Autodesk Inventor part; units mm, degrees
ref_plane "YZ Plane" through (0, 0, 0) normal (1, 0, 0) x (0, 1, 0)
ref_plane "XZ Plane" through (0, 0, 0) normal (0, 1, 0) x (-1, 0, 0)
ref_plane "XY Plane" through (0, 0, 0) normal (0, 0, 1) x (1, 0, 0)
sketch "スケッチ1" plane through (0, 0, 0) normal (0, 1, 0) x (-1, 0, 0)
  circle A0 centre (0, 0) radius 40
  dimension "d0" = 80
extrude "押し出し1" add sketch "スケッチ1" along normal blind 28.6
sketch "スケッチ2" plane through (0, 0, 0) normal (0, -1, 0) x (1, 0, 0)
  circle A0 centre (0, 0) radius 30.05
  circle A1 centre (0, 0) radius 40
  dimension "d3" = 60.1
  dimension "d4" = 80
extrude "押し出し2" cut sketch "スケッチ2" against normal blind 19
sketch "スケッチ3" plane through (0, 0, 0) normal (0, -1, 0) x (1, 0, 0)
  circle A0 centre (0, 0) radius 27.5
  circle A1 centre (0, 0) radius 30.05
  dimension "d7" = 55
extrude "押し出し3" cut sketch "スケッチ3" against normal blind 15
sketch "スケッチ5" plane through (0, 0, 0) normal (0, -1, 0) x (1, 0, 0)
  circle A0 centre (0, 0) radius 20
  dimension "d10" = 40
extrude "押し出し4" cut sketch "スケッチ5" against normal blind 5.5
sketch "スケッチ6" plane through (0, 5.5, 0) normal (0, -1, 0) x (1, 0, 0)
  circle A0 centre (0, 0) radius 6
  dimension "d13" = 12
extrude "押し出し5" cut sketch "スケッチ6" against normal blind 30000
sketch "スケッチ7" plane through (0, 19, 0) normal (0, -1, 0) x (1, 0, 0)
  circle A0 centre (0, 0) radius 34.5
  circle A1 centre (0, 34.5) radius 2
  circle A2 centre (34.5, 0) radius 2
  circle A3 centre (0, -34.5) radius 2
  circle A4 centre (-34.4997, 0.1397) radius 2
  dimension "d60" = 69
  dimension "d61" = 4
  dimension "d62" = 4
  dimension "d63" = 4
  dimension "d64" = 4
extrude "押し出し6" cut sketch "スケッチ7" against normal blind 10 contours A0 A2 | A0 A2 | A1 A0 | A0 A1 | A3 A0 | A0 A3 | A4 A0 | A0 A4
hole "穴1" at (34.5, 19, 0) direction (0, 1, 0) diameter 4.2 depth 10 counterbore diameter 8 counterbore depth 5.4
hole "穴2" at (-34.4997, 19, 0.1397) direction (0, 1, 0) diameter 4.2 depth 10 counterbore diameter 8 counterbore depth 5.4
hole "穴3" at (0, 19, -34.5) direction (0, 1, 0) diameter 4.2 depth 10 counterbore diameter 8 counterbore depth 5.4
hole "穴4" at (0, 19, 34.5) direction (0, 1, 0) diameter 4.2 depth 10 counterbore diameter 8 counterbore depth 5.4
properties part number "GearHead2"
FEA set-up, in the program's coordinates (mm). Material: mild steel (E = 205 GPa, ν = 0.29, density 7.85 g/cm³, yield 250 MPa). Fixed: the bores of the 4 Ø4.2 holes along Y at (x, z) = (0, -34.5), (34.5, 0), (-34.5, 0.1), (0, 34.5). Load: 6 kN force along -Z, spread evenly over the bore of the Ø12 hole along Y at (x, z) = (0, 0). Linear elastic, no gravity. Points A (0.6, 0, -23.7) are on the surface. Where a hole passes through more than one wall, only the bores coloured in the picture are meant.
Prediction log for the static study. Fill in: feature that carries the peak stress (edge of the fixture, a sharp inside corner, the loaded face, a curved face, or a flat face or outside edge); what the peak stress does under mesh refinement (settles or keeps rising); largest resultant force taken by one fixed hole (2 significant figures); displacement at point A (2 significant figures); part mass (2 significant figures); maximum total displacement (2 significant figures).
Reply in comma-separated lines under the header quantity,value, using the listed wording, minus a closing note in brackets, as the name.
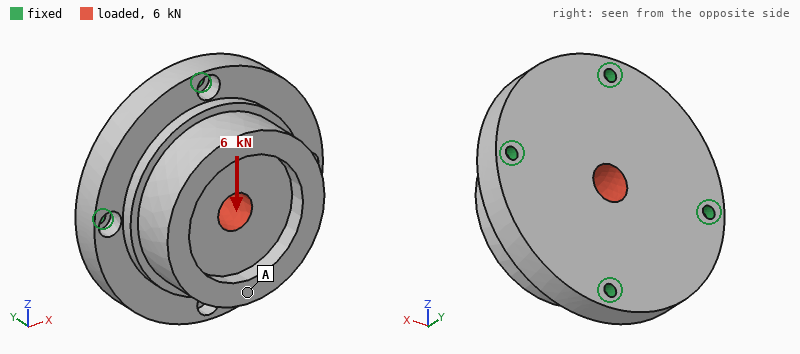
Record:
quantity,value
feature that carries the peak stress,edge of the fixture
what the peak stress does under mesh refinement,keeps rising
largest resultant force taken by one fixed hole,2.0 kN
displacement at point A,2.2 µm
part mass,660 g
maximum total displacement,2.3 µm
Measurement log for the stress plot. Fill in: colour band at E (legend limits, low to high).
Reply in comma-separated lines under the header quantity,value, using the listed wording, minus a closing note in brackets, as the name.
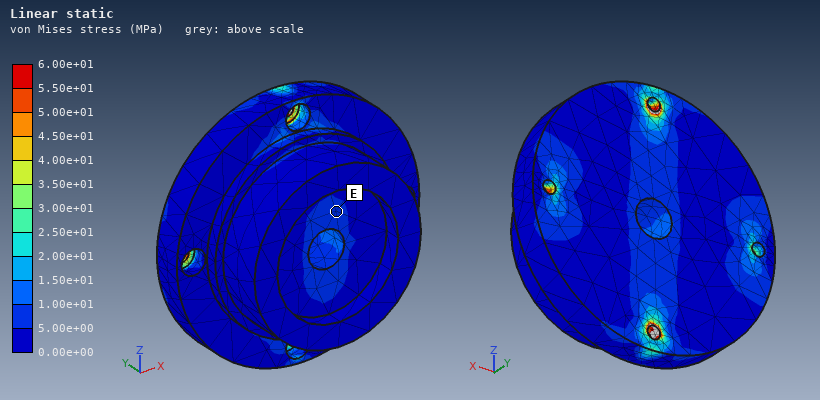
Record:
quantity,value
colour band at E,5.00e+00 to 1.00e+01 MPa
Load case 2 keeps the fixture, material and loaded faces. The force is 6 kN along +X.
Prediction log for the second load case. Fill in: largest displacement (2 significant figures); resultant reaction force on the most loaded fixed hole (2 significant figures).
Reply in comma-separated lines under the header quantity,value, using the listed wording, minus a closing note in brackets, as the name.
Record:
quantity,value
largest displacement,2.3 µm
resultant reaction force on the most loaded fixed hole,2.0 kN
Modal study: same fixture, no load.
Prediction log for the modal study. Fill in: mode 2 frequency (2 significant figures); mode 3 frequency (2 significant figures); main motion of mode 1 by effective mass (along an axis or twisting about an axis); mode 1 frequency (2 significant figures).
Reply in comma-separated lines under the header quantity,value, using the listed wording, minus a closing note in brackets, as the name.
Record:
quantity,value
mode 2 frequency,11 kHz
mode 3 frequency,11 kHz
main motion of mode 1 by effective mass,along Y
mode 1 frequency,9800 Hz
